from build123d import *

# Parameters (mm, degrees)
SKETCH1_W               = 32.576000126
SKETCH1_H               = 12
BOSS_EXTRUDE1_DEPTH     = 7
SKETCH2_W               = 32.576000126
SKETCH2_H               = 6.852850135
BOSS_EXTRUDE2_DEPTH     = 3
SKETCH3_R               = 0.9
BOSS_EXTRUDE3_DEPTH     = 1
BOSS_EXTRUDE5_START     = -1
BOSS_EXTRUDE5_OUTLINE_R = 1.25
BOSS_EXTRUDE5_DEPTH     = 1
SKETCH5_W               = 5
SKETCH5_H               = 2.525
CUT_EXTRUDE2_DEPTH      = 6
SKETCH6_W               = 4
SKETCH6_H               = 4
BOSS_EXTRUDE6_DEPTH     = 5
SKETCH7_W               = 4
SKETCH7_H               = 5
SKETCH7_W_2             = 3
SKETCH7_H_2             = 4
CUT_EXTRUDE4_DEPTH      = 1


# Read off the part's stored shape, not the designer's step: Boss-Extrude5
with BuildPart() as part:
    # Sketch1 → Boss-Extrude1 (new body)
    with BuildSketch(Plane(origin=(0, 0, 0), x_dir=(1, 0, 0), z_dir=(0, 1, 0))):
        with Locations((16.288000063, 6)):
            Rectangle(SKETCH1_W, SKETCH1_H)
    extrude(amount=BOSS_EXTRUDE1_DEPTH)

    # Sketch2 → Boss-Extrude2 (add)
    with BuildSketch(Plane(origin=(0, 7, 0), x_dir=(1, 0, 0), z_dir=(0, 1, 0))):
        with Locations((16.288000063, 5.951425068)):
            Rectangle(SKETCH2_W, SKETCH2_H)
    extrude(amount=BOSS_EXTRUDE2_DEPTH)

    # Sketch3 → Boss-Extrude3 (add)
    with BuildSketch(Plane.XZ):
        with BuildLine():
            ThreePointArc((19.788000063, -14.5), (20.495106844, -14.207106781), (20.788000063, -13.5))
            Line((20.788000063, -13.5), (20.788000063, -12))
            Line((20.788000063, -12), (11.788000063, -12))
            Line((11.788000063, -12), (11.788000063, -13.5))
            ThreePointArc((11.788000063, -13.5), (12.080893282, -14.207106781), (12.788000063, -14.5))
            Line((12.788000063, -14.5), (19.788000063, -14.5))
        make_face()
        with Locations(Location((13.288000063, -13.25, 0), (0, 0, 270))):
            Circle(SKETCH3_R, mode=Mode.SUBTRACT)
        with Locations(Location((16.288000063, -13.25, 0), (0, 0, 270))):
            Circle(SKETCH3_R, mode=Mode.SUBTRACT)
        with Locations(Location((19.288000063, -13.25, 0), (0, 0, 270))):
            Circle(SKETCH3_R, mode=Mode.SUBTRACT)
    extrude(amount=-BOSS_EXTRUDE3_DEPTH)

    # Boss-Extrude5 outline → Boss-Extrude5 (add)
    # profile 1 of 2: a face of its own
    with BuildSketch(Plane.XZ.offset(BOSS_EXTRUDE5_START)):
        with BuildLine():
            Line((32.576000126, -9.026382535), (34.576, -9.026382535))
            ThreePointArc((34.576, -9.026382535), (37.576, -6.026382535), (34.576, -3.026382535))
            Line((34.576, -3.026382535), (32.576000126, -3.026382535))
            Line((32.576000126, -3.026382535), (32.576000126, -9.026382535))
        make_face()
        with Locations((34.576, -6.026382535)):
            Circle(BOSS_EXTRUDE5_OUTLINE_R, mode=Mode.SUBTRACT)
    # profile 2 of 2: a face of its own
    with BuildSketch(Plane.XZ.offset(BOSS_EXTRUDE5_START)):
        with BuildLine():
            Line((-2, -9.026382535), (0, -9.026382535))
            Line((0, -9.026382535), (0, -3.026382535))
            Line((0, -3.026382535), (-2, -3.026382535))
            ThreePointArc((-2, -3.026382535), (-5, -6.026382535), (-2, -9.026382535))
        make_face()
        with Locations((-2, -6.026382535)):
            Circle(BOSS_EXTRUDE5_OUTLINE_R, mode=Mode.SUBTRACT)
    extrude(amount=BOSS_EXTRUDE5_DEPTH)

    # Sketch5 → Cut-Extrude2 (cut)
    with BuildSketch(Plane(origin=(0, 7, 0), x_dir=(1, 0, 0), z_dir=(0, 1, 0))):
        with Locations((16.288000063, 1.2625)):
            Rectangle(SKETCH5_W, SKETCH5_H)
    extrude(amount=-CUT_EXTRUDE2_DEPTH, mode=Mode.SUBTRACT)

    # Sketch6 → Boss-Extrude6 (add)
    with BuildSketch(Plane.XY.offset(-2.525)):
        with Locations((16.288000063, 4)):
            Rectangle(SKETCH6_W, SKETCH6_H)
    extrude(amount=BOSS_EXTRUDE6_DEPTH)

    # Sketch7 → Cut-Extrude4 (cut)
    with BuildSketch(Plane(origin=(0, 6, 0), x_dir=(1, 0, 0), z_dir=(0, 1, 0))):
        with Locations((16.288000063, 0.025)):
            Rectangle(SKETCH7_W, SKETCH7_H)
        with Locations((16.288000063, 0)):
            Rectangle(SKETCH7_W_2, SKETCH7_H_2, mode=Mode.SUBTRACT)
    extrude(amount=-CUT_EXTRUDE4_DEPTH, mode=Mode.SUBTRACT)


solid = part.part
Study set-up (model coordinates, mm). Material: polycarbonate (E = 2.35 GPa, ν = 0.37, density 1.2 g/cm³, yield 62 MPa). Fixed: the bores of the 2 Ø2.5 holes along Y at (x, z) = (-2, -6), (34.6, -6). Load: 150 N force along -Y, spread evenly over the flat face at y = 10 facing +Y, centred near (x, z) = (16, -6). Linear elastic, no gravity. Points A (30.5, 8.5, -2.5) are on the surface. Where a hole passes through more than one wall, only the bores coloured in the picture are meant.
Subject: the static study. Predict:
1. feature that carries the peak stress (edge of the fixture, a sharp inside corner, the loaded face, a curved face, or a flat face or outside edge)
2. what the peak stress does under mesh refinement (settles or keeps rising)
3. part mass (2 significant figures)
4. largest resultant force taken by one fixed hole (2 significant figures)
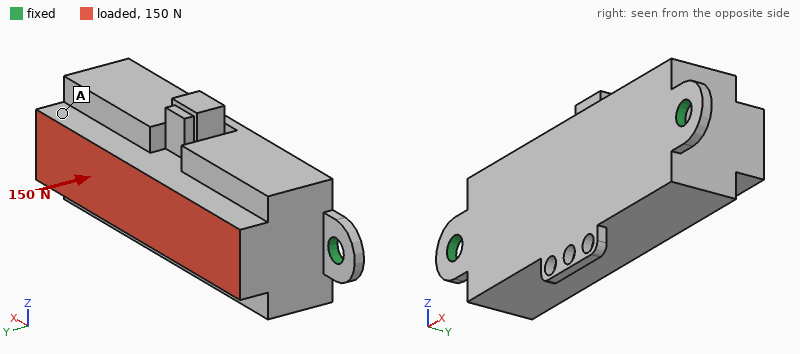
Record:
edge of the fixture
keeps rising
4.2 g
94 N
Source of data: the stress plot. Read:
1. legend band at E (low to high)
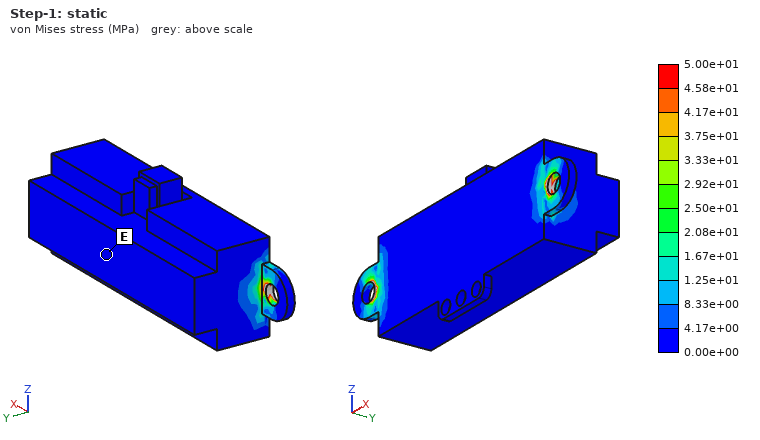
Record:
0.00e+00 to 4.17e+00 MPa
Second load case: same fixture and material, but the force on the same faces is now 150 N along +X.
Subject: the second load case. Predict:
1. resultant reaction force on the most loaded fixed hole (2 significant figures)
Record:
86 N
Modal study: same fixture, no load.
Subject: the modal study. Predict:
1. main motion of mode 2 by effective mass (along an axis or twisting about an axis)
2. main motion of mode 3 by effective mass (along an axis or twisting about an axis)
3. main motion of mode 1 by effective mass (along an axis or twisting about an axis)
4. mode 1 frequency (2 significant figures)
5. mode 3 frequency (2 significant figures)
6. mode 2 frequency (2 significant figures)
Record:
along Y
along Z
along Z
920 Hz
4800 Hz
3400 Hz
